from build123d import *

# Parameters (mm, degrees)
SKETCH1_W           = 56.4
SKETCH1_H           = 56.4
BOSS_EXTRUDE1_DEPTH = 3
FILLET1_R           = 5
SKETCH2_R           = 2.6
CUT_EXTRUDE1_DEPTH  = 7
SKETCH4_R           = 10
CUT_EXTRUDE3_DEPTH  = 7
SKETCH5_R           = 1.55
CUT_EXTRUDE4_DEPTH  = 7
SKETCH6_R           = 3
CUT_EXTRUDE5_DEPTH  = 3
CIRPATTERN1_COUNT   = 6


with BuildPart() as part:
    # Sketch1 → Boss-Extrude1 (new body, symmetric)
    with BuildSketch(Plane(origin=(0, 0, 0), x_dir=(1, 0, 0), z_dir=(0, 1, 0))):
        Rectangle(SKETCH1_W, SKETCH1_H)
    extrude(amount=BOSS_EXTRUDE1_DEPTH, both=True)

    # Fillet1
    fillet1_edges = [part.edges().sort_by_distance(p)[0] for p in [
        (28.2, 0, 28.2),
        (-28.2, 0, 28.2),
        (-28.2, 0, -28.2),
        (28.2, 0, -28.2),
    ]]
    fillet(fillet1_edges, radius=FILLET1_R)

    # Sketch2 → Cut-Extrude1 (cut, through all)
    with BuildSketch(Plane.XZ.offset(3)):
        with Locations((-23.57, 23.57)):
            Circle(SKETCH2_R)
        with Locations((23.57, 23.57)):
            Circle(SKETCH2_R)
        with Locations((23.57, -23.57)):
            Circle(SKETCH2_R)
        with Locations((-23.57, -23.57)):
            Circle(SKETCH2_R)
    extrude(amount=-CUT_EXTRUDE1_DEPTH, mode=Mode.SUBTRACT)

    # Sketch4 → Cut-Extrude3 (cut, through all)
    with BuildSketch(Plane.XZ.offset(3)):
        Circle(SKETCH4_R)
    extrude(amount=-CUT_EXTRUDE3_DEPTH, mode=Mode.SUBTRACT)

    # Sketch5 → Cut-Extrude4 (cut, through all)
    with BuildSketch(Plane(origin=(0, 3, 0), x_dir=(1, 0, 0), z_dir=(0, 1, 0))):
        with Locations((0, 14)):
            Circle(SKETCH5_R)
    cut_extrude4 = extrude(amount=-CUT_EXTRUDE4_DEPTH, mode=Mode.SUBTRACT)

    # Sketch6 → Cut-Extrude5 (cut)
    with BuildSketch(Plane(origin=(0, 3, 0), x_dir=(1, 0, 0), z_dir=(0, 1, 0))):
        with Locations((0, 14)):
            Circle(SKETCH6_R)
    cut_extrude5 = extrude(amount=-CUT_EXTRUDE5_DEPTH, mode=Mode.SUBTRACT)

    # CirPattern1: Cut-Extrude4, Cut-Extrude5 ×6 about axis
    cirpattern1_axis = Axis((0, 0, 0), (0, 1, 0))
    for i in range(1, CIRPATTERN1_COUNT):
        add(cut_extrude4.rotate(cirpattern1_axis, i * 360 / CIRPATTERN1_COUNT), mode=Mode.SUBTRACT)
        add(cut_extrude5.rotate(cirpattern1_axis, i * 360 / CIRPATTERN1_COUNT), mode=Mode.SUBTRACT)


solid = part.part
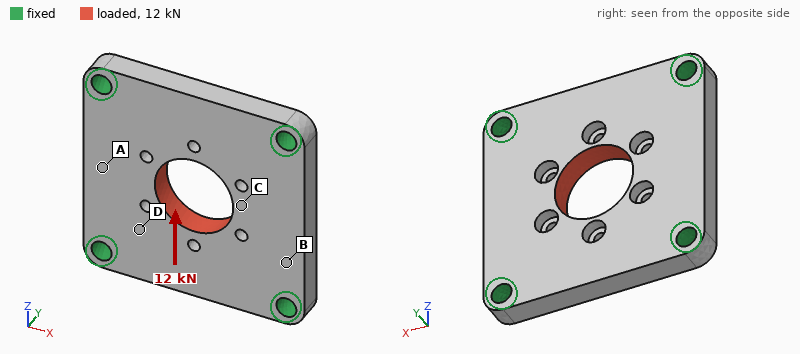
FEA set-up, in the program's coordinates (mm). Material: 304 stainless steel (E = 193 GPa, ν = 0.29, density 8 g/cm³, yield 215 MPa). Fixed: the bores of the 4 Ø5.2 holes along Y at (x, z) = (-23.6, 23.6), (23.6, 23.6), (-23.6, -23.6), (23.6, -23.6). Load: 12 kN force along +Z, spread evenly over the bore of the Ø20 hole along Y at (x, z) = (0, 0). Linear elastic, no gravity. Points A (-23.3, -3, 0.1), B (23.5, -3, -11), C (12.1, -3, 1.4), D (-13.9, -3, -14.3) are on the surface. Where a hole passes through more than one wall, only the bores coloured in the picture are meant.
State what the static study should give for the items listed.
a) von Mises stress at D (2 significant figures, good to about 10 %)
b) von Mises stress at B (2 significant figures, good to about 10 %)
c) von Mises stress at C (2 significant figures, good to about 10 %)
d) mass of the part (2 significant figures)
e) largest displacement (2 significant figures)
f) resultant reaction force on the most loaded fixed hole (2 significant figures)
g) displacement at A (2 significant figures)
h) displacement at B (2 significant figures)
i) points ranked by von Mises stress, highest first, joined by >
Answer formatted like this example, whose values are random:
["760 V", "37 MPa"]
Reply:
["39 MPa", "24 MPa", "65 MPa", "130 g", "10 µm", "3.3 kN", "2.2 µm", "1.7 µm", "C > D > B > A"]
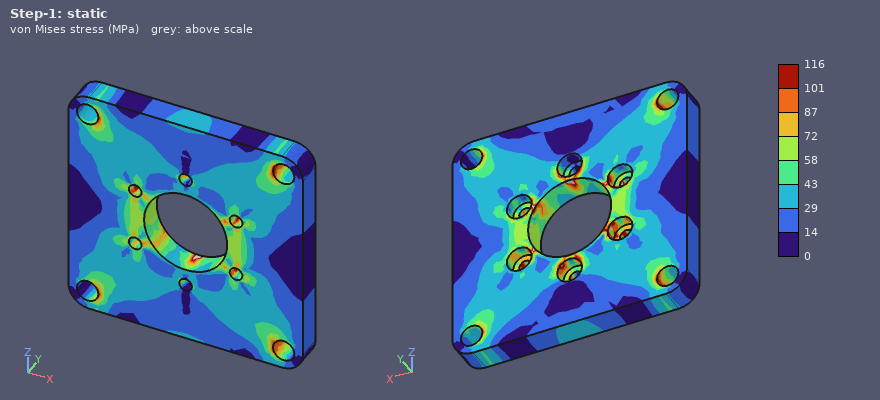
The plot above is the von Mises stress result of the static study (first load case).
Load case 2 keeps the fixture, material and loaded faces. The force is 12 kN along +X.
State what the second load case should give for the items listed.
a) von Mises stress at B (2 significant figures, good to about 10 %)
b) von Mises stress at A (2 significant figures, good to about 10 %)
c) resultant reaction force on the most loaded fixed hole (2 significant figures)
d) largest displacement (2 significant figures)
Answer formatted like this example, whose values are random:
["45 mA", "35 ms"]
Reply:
["23 MPa", "18 MPa", "3.3 kN", "9.6 µm"]
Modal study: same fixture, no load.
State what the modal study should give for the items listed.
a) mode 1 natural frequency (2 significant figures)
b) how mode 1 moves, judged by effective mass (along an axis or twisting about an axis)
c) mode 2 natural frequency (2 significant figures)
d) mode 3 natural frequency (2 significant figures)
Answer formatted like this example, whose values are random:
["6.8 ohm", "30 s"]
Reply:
["9600 Hz", "along Y", "14 kHz", "14 kHz"]
